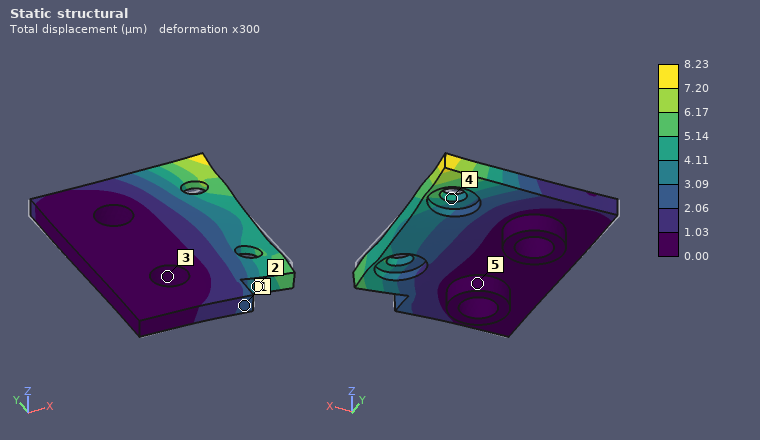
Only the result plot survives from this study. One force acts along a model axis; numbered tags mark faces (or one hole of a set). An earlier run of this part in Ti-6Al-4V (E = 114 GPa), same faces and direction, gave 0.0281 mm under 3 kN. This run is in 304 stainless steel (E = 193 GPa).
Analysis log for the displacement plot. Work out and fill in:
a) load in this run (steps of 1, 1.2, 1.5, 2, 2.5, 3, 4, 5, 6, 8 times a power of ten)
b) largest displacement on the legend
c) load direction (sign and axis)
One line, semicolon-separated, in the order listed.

1.5 kN; 8.23 µm; -Y
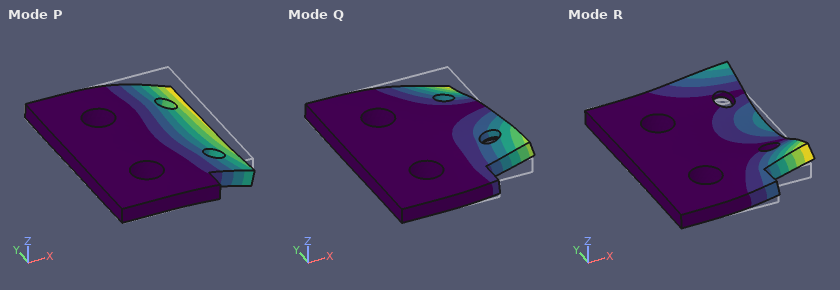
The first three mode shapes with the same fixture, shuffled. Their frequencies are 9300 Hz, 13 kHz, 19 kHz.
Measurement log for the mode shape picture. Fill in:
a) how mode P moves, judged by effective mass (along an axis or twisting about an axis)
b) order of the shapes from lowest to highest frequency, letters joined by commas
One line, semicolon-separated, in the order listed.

along Z; P, Q, R
